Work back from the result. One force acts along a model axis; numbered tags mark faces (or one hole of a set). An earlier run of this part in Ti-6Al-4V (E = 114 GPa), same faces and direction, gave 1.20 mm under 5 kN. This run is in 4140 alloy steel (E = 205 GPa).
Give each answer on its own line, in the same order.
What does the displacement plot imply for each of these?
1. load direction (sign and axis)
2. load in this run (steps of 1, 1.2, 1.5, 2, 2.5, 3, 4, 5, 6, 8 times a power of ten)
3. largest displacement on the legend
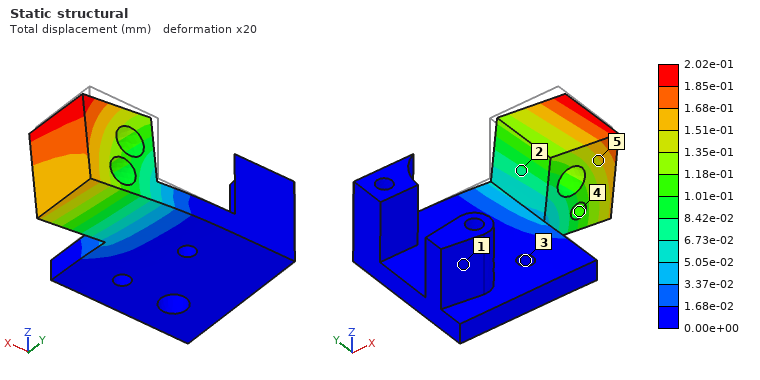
-Z
1.5 kN
2.02e-01 mm
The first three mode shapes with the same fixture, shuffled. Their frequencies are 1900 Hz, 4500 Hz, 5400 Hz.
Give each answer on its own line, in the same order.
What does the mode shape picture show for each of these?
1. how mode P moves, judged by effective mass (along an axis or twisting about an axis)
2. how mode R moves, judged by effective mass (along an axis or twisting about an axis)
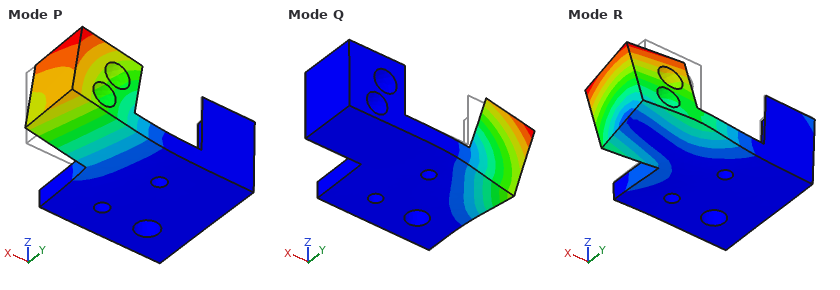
along Z
along Y
